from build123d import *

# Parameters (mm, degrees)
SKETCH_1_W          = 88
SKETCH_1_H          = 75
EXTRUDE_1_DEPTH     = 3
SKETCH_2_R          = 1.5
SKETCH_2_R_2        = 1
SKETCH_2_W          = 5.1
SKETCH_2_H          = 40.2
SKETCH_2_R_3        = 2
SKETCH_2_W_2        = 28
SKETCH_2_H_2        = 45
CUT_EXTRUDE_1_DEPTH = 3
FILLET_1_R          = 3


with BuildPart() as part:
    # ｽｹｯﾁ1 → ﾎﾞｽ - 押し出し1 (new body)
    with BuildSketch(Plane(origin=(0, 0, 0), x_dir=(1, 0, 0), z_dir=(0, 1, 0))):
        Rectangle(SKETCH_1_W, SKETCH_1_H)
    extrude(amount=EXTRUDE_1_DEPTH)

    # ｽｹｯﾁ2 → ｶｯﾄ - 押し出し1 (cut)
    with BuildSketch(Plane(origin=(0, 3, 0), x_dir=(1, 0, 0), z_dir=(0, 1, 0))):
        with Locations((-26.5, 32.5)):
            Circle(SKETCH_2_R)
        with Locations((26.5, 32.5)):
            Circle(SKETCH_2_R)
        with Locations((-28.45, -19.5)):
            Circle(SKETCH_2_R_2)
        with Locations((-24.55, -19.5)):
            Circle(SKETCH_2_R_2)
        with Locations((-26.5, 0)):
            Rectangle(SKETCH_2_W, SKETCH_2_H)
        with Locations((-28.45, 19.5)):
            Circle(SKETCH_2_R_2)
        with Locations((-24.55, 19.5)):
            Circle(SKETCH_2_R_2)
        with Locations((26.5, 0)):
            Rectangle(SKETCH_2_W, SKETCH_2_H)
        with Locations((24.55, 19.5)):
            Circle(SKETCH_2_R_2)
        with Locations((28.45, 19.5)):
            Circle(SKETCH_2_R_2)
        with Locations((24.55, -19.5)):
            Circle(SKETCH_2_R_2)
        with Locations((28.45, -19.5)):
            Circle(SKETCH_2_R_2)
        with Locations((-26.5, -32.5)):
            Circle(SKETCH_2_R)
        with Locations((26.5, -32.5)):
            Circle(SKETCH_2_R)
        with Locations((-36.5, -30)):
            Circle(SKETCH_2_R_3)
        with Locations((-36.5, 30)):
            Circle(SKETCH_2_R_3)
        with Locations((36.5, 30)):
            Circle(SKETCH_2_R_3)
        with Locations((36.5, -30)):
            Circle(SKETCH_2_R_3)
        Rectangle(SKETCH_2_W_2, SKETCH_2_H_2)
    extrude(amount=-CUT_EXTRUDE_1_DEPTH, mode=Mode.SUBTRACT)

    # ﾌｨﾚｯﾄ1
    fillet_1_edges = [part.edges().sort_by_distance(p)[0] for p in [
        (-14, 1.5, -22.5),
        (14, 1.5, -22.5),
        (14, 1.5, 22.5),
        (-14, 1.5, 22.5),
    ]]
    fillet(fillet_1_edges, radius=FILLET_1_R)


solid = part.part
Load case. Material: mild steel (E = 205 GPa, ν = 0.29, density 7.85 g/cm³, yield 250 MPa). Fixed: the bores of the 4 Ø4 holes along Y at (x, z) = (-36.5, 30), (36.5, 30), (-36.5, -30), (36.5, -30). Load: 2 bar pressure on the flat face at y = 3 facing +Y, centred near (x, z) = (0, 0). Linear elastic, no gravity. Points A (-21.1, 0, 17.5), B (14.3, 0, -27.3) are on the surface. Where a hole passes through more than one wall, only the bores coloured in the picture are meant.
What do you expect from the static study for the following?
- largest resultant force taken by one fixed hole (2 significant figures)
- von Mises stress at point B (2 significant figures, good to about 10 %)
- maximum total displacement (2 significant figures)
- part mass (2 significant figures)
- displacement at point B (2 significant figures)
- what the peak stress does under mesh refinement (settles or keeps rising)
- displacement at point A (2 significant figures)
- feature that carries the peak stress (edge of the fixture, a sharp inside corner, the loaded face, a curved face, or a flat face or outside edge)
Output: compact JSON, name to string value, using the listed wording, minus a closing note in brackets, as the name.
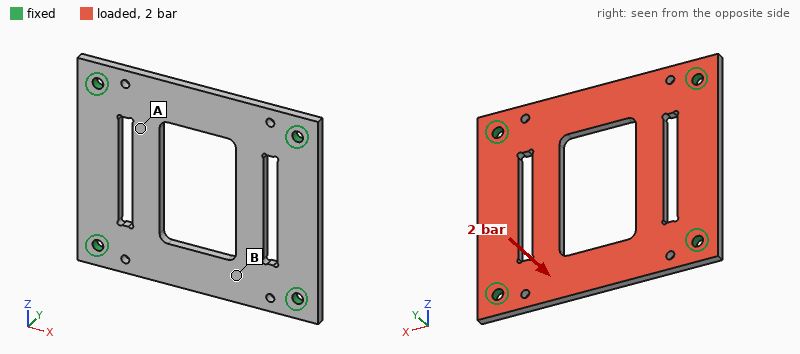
{"largest resultant force taken by one fixed hole": "240 N", "von Mises stress at point B": "21 MPa", "maximum total displacement": "50 µm", "part mass": "110 g", "displacement at point B": "29 µm", "what the peak stress does under mesh refinement": "keeps rising", "displacement at point A": "27 µm", "feature that carries the peak stress": "edge of the fixture"}
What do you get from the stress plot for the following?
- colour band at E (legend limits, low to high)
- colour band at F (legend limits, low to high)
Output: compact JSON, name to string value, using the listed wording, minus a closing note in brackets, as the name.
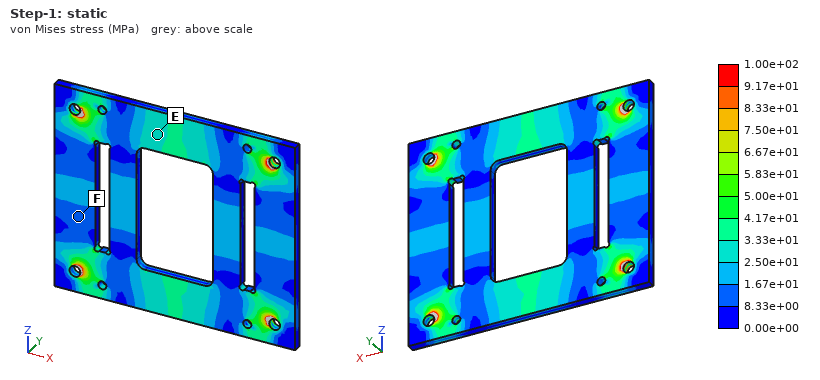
{"colour band at E": "2.50e+01 to 3.33e+01 MPa", "colour band at F": "8.33e+00 to 1.67e+01 MPa"}
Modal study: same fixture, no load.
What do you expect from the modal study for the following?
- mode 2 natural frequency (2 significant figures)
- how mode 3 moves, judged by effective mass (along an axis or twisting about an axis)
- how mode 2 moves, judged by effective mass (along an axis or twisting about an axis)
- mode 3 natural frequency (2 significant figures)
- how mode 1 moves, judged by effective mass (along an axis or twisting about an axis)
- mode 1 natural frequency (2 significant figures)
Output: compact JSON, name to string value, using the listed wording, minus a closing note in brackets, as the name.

{"mode 2 natural frequency": "3400 Hz", "how mode 3 moves, judged by effective mass": "twisting about Z", "how mode 2 moves, judged by effective mass": "twisting about X", "mode 3 natural frequency": "3900 Hz", "how mode 1 moves, judged by effective mass": "along Y", "mode 1 natural frequency": "2600 Hz"}
